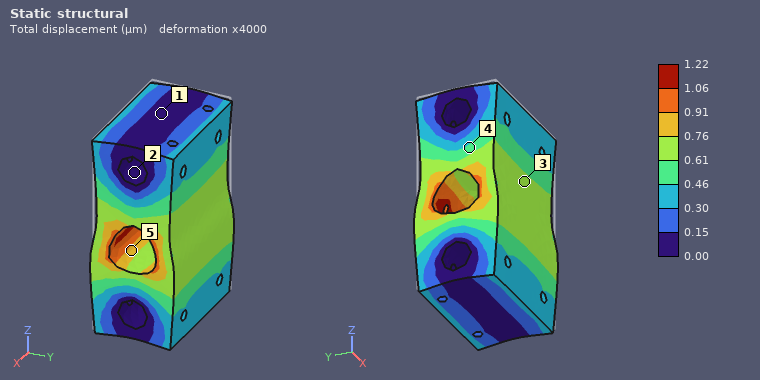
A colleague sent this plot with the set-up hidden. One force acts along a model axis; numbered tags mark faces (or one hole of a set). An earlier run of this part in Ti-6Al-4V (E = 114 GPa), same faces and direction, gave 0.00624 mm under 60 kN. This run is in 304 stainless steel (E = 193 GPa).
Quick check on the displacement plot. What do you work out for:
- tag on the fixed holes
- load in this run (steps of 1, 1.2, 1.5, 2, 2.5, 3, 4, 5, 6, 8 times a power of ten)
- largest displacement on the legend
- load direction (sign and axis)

2
20 kN
1.22 µm
-Z
